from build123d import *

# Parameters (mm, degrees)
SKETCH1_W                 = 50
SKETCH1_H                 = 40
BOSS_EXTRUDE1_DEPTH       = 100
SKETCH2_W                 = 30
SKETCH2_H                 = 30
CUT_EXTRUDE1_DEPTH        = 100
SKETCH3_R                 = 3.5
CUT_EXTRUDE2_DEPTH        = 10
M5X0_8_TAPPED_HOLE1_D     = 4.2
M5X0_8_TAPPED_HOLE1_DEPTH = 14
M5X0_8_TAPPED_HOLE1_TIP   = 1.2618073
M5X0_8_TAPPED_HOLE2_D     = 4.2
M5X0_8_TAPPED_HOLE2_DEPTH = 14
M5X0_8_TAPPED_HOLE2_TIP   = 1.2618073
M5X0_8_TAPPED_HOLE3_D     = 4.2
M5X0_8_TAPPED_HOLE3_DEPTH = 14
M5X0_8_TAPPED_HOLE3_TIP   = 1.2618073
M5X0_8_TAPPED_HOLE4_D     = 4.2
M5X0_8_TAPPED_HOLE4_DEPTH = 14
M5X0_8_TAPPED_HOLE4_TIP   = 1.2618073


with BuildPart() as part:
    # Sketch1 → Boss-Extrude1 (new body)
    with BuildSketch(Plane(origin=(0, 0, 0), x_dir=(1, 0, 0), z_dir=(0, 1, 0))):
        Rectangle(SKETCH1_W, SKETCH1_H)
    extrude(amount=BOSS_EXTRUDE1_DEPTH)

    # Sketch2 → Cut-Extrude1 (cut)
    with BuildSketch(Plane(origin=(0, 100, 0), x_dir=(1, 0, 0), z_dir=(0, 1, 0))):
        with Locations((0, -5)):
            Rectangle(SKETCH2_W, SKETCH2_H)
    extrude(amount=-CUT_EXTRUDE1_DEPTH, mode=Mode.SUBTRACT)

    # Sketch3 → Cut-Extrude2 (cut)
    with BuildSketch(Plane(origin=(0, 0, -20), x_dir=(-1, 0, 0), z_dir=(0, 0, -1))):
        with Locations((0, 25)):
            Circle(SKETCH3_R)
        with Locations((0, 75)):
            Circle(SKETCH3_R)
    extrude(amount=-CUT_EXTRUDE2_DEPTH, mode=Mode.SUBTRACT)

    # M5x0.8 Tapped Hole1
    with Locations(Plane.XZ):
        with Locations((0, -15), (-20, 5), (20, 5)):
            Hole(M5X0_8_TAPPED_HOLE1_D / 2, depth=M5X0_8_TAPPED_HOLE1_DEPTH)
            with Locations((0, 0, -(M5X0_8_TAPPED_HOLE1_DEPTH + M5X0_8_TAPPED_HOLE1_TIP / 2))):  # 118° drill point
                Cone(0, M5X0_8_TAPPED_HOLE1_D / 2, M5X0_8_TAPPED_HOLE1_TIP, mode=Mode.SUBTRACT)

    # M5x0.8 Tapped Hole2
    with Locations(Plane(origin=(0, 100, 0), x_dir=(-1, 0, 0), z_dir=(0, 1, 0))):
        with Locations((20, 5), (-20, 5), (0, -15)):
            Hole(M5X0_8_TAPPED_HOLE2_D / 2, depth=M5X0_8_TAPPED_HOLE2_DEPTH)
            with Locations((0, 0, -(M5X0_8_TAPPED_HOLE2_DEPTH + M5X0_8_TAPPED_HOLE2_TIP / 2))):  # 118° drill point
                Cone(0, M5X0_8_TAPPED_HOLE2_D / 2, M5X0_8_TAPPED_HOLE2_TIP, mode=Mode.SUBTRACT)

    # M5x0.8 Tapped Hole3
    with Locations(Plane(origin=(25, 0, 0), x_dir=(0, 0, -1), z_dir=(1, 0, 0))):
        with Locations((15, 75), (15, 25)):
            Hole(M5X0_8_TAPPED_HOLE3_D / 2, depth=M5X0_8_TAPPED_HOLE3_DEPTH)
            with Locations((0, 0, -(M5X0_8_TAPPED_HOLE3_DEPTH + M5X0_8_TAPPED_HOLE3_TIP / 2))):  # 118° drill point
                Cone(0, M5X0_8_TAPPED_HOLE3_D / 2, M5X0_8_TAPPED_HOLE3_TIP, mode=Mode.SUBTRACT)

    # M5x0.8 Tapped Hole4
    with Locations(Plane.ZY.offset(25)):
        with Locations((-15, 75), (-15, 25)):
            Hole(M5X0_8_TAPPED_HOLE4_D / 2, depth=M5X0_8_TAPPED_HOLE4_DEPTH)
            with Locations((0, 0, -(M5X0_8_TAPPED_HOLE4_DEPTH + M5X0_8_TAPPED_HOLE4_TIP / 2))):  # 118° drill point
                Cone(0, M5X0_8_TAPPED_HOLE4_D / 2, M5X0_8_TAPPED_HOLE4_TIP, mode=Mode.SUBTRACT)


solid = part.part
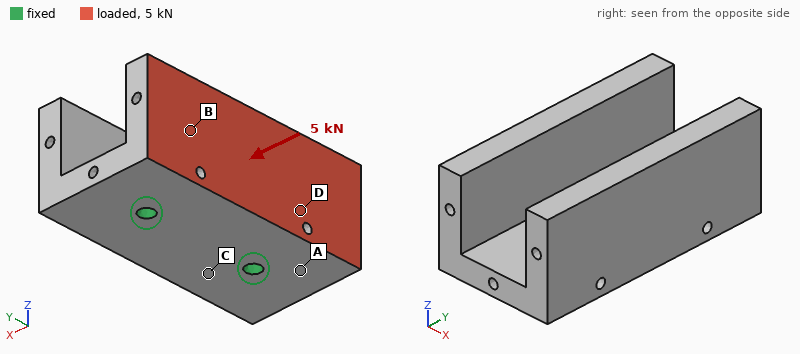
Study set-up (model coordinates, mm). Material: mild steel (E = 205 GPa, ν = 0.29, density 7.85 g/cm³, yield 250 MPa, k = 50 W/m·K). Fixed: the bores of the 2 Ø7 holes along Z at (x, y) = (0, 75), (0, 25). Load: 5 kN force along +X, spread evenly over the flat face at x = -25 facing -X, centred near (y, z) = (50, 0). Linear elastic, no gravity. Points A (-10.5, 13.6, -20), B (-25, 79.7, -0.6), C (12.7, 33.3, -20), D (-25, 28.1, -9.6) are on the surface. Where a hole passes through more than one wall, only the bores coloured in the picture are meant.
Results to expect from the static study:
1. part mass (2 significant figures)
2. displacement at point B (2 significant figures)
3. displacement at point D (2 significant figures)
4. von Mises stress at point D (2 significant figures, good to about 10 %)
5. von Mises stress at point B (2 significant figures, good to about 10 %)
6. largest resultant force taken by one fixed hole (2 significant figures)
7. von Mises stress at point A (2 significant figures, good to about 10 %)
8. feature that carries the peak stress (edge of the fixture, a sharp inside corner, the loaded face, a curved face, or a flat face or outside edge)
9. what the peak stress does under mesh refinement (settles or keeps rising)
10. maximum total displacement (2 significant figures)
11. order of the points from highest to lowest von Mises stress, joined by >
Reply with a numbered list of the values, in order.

1. 840 g
2. 25 µm
3. 18 µm
4. 28 MPa
5. 16 MPa
6. 2.5 kN
7. 35 MPa
8. edge of the fixture
9. keeps rising
10. 49 µm
11. A > D > B > C
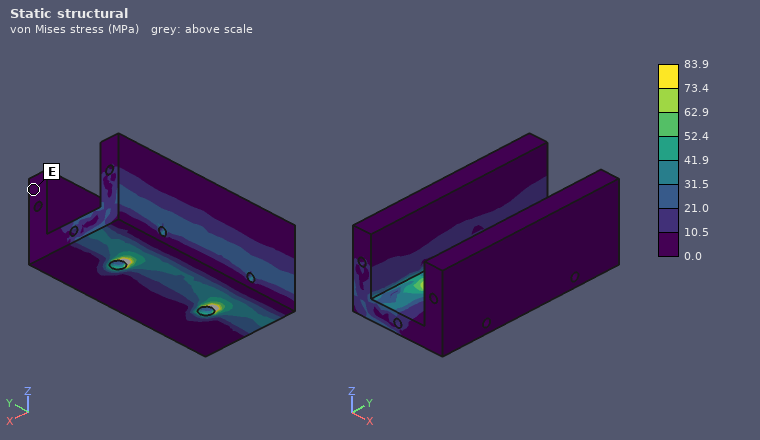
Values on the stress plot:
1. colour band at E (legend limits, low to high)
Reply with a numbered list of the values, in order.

1. 0.0 to 10.5 MPa
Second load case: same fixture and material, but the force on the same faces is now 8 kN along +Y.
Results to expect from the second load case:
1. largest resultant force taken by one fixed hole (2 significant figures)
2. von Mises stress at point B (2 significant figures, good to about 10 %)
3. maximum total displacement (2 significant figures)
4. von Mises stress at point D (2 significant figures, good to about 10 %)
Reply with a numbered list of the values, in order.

1. 5.7 kN
2. 10 MPa
3. 17 µm
4. 11 MPa
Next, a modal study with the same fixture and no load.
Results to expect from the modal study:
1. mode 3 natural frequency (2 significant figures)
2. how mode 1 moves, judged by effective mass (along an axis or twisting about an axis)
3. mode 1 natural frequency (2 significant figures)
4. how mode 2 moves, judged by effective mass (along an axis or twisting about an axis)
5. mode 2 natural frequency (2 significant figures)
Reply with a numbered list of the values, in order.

1. 4500 Hz
2. along X
3. 2900 Hz
4. along Z
5. 3700 Hz
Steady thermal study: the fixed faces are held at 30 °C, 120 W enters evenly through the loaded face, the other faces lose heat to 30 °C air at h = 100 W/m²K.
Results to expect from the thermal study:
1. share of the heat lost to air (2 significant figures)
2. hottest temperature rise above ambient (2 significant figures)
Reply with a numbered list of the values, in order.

1. 42 %
2. 64 K
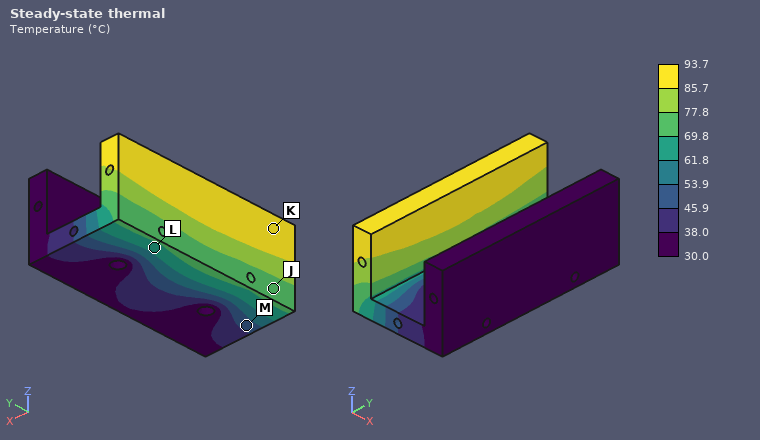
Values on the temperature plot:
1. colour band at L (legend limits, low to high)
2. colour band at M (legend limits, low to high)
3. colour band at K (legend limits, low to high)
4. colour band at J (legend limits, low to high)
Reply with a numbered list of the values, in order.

1. 61.8 to 69.8 °C
2. 45.9 to 53.9 °C
3. 85.7 to 93.7 °C
4. 69.8 to 77.8 °C
